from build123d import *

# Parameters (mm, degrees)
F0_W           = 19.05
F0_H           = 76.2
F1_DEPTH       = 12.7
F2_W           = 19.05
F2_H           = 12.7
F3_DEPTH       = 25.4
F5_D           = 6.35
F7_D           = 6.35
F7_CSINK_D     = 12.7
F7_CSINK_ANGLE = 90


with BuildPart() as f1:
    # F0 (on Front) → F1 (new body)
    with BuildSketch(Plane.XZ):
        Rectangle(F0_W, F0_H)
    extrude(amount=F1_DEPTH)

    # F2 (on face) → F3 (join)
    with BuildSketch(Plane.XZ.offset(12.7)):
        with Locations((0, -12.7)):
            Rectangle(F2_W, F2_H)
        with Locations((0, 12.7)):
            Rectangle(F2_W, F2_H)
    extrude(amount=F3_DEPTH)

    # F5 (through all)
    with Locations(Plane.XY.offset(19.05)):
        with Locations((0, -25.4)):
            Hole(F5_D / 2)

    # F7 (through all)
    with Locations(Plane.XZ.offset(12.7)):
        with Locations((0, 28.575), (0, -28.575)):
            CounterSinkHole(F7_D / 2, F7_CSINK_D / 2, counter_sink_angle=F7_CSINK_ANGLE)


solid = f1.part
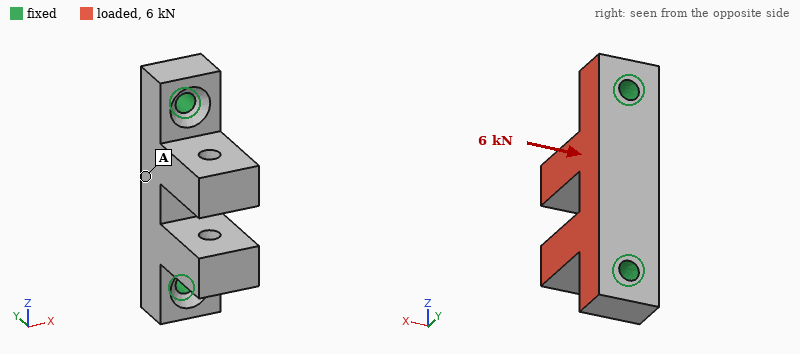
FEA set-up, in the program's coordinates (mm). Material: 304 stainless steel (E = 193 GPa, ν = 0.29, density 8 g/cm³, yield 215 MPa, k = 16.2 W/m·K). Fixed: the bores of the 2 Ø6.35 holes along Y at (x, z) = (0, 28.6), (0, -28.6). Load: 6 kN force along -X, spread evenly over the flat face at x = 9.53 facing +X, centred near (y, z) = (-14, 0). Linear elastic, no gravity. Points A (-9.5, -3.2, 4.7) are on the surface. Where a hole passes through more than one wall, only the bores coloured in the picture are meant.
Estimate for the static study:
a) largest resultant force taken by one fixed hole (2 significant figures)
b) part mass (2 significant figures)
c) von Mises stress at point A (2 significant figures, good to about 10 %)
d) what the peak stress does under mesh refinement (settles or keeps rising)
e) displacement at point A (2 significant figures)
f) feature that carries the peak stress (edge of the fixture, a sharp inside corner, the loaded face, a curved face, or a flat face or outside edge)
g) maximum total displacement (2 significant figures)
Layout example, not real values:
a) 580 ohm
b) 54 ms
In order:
a) 3.0 kN
b) 230 g
c) 22 MPa
d) keeps rising
e) 6.7 µm
f) edge of the fixture
g) 30 µm
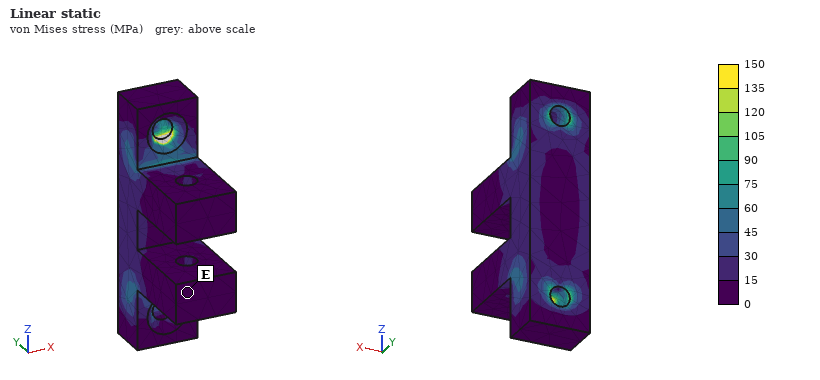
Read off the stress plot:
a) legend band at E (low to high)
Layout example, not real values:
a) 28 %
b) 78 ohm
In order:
a) 0 to 15 MPa
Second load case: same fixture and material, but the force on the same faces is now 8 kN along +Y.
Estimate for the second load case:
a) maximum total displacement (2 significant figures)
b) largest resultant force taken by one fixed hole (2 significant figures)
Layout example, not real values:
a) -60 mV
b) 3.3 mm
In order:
a) 36 µm
b) 4.1 kN
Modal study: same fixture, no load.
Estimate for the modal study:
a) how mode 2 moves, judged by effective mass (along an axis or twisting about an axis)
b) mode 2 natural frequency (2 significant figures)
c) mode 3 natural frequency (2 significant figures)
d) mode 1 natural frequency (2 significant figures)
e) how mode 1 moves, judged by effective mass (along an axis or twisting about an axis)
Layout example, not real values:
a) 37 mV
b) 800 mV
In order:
a) along Y
b) 7100 Hz
c) 8700 Hz
d) 5700 Hz
e) along X
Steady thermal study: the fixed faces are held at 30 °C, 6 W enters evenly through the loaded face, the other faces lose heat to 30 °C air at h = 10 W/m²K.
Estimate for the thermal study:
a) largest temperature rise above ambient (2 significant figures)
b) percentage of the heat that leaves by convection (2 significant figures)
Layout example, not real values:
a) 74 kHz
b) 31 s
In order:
a) 13 K
b) 8.6 %
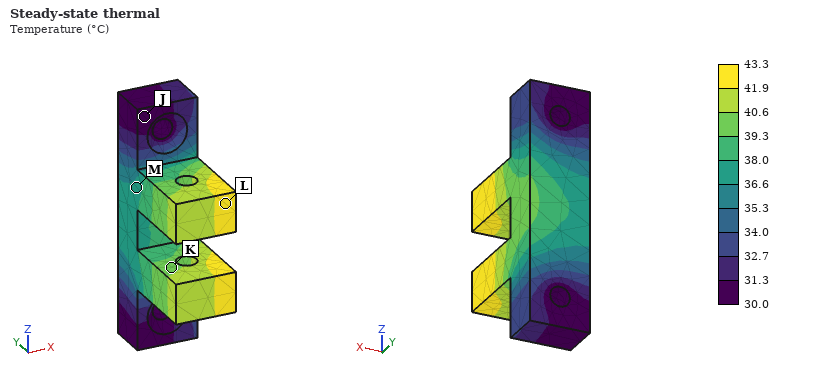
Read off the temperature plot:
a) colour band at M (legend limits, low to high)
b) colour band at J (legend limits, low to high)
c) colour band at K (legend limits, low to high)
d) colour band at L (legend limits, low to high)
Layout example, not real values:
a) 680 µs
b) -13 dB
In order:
a) 36.6 to 38.0 °C
b) 30.0 to 31.3 °C
c) 39.3 to 40.6 °C
d) 41.9 to 43.3 °C
